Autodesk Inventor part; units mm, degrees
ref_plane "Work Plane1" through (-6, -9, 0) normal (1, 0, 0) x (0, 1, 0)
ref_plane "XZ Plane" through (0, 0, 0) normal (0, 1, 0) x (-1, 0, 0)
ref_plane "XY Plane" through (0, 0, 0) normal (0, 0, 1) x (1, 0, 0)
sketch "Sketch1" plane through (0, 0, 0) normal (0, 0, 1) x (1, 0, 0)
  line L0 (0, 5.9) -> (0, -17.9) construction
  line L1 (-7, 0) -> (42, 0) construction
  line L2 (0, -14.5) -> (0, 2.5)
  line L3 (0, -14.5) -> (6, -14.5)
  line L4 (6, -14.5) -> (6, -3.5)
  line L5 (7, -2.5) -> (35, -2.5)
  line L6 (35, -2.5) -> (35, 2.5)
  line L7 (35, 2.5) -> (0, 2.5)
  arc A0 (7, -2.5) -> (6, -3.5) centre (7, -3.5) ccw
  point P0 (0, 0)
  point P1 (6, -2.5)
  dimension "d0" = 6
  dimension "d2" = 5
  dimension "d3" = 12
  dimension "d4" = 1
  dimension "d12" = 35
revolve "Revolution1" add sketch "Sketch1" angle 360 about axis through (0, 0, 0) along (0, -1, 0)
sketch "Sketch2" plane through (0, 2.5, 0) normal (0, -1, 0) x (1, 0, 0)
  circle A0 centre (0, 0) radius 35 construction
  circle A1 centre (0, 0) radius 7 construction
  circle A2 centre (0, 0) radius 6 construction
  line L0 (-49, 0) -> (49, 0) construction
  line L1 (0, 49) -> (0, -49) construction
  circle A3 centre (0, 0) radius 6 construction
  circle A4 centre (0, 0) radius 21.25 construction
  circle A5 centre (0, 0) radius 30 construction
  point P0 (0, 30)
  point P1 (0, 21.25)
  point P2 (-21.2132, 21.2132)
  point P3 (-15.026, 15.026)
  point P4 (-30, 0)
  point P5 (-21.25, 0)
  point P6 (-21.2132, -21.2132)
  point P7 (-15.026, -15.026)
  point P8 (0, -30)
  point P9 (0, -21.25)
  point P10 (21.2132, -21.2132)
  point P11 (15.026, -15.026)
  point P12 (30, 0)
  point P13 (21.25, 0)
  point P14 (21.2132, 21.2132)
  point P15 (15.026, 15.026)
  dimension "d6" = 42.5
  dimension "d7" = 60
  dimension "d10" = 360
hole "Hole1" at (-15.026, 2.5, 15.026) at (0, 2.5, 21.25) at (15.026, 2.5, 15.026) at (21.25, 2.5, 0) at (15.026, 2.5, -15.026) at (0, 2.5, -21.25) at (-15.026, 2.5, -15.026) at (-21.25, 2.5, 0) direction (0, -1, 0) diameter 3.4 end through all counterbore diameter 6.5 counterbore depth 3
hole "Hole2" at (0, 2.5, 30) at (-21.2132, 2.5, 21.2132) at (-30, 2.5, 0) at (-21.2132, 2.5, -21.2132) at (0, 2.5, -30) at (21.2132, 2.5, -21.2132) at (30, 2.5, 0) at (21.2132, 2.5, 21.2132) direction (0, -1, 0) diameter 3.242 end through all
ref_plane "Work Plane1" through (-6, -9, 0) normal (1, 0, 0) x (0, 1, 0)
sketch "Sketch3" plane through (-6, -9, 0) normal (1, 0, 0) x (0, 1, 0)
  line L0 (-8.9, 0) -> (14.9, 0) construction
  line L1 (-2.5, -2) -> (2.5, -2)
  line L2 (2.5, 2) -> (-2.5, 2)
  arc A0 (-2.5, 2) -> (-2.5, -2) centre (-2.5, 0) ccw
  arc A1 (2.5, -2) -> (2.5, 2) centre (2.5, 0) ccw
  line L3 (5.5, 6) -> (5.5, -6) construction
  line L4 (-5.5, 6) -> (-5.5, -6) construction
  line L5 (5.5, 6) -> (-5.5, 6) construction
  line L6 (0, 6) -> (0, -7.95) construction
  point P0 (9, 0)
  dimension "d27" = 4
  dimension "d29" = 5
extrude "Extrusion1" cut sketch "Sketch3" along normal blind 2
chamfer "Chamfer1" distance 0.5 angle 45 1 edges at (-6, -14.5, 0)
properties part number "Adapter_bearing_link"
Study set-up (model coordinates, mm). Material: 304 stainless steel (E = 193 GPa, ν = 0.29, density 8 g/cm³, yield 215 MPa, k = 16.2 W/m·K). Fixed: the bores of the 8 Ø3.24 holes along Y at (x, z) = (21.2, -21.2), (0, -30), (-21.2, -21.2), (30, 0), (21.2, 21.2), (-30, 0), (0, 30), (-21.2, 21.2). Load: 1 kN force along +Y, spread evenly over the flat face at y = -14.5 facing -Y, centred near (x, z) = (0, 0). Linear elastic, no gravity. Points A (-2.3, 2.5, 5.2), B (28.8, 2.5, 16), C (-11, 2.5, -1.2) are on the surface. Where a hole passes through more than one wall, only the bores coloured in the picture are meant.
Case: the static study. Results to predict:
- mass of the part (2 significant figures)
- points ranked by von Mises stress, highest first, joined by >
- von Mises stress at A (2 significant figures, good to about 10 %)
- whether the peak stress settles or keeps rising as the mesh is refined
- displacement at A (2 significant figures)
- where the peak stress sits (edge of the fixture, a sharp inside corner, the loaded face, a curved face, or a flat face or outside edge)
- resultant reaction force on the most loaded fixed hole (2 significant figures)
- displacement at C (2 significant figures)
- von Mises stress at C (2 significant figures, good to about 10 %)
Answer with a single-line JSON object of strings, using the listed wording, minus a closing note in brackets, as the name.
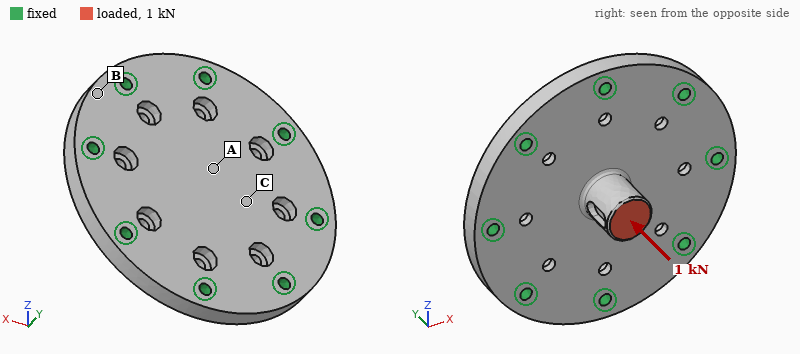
{"mass of the part": "150 g", "points ranked by von Mises stress, highest first, joined by >": "A > C > B", "von Mises stress at A": "27 MPa", "whether the peak stress settles or keeps rising as the mesh is refined": "keeps rising", "displacement at A": "7.7 µm", "where the peak stress sits": "edge of the fixture", "resultant reaction force on the most loaded fixed hole": "130 N", "displacement at C": "6.1 µm", "von Mises stress at C": "18 MPa"}
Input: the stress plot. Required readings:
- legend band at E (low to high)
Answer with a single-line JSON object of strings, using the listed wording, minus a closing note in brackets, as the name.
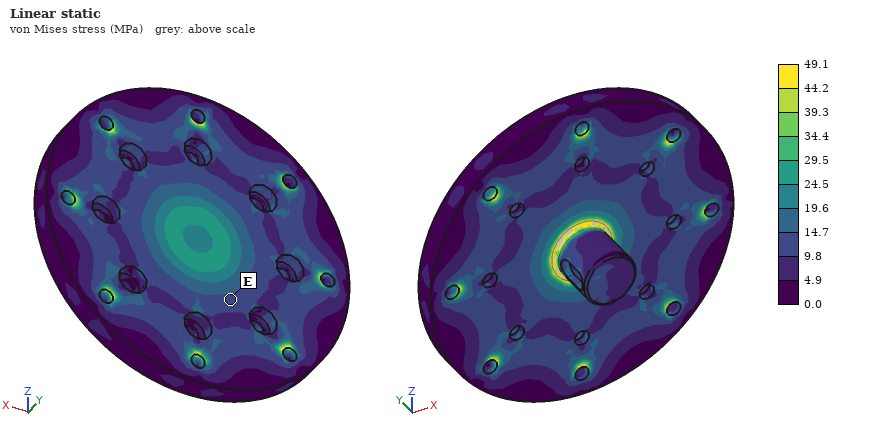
{"legend band at E": "9.8 to 14.7 MPa"}
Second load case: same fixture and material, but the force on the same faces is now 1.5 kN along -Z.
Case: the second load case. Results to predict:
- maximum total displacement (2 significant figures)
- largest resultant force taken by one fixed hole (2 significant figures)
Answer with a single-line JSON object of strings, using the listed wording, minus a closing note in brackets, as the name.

{"maximum total displacement": "24 µm", "largest resultant force taken by one fixed hole": "390 N"}
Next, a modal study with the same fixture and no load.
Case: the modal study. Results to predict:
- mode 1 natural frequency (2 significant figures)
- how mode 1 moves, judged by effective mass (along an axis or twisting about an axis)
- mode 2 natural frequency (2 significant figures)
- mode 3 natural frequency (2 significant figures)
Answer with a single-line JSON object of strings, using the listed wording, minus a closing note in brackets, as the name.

{"mode 1 natural frequency": "9400 Hz", "how mode 1 moves, judged by effective mass": "along Y", "mode 2 natural frequency": "16 kHz", "mode 3 natural frequency": "16 kHz"}
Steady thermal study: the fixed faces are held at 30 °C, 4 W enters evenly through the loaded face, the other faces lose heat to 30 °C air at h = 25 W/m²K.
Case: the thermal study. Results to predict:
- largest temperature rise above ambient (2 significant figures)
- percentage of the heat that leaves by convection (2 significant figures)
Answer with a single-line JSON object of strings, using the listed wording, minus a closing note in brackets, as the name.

{"largest temperature rise above ambient": "44 K", "percentage of the heat that leaves by convection": "25 %"}
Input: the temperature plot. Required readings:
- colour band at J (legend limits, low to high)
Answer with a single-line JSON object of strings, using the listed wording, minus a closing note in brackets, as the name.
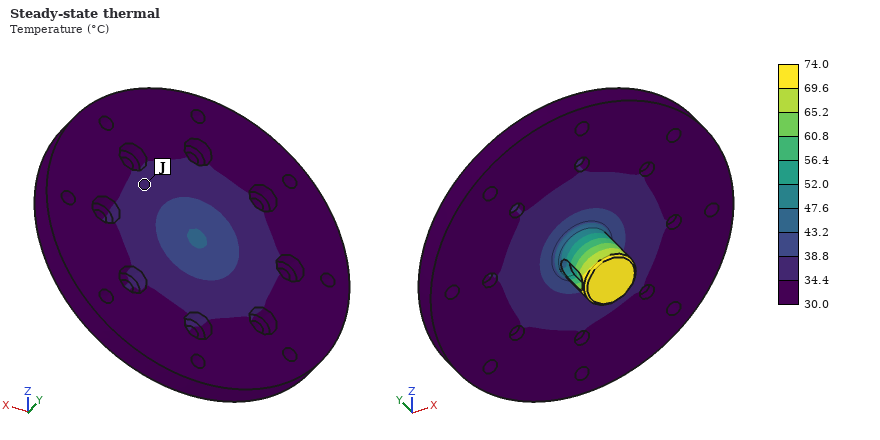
{"colour band at J": "34.4 to 38.8 °C"}
